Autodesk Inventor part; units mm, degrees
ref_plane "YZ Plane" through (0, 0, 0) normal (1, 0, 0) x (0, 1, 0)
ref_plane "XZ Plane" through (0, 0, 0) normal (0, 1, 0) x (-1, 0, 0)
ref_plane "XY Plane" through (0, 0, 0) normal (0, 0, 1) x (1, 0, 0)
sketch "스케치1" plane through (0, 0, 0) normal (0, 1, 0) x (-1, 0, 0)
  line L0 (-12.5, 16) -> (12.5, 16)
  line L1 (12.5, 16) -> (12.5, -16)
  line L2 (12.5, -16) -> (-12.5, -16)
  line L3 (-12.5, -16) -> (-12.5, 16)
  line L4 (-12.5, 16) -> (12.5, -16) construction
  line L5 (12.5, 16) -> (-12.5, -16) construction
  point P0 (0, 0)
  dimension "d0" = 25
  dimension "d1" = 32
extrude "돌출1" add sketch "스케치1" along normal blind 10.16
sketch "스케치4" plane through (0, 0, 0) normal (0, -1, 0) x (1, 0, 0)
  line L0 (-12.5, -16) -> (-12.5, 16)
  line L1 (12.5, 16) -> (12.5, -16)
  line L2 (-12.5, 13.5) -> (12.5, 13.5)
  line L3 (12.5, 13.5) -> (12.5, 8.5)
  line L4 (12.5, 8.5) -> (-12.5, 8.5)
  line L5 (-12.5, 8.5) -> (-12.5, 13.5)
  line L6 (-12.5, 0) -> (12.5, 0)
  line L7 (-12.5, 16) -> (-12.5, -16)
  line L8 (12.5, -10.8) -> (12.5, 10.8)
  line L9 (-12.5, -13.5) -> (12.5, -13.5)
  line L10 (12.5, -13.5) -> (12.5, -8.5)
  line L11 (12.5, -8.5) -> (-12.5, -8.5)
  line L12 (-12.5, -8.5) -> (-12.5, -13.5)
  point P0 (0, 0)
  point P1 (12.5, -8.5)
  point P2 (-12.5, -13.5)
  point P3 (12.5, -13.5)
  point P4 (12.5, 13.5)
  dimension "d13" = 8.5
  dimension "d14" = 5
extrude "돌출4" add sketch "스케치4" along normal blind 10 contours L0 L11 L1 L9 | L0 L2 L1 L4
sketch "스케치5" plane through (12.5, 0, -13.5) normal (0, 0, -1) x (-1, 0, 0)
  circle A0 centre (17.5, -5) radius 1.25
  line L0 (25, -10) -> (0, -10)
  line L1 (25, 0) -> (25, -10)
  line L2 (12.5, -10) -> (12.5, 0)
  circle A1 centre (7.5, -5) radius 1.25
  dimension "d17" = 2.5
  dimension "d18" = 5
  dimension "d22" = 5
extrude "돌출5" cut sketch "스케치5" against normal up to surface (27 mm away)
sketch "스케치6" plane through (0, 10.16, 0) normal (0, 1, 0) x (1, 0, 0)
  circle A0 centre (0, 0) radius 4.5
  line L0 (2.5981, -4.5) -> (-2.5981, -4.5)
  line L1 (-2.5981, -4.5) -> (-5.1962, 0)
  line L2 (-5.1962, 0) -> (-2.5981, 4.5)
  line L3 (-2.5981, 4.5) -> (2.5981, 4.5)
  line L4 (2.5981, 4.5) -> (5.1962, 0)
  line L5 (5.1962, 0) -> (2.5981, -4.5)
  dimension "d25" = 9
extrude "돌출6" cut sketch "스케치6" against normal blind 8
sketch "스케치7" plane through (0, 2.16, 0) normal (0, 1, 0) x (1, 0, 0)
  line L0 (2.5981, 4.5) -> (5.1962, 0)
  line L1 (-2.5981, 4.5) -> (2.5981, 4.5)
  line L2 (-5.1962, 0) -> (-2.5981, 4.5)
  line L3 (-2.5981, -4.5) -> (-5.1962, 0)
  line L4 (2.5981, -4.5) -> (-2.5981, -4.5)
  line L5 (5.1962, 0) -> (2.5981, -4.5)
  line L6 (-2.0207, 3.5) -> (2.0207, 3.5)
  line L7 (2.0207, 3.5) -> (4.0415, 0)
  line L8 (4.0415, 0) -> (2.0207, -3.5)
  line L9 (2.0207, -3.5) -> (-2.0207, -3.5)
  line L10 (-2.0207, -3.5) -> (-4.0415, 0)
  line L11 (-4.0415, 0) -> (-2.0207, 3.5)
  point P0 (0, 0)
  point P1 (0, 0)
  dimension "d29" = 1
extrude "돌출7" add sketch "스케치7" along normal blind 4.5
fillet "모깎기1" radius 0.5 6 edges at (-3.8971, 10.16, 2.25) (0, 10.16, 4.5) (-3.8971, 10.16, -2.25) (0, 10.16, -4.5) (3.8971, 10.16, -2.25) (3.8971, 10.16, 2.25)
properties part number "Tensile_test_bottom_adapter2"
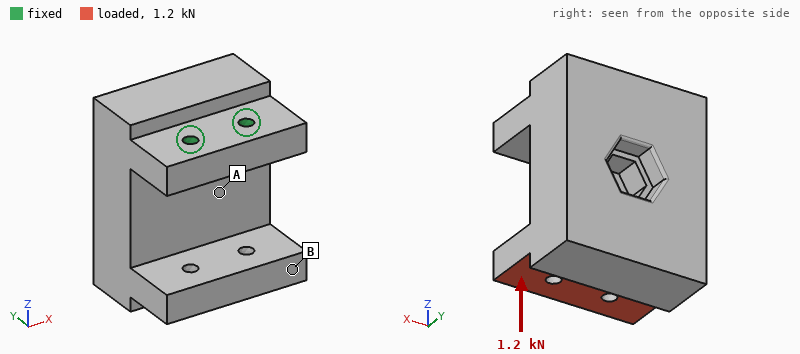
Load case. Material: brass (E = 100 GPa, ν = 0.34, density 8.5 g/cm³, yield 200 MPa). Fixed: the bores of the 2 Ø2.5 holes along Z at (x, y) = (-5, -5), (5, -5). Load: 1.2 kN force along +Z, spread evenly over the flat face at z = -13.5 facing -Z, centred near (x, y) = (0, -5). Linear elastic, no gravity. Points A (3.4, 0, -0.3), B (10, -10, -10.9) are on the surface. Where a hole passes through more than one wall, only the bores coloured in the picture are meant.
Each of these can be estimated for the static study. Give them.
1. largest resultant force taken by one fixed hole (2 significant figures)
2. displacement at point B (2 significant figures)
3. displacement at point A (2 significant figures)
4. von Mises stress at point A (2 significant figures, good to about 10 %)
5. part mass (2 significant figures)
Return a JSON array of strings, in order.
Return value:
["600 N", "54 µm", "15 µm", "36 MPa", "86 g"]
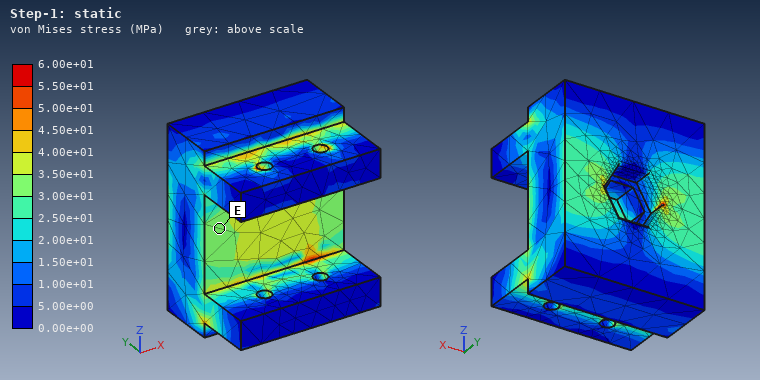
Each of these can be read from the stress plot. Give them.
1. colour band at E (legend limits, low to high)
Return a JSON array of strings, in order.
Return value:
["3.00e+01 to 3.50e+01 MPa"]
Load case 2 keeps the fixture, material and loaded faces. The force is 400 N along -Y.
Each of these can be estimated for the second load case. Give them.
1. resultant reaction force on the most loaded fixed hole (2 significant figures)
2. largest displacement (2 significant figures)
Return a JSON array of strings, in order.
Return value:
["200 N", "93 µm"]
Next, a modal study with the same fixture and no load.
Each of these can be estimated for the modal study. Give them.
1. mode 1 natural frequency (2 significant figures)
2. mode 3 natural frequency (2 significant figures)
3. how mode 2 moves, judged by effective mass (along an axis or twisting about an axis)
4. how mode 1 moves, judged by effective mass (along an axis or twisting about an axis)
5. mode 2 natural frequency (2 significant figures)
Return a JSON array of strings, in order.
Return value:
["1900 Hz", "7600 Hz", "along X", "along Y", "3500 Hz"]
